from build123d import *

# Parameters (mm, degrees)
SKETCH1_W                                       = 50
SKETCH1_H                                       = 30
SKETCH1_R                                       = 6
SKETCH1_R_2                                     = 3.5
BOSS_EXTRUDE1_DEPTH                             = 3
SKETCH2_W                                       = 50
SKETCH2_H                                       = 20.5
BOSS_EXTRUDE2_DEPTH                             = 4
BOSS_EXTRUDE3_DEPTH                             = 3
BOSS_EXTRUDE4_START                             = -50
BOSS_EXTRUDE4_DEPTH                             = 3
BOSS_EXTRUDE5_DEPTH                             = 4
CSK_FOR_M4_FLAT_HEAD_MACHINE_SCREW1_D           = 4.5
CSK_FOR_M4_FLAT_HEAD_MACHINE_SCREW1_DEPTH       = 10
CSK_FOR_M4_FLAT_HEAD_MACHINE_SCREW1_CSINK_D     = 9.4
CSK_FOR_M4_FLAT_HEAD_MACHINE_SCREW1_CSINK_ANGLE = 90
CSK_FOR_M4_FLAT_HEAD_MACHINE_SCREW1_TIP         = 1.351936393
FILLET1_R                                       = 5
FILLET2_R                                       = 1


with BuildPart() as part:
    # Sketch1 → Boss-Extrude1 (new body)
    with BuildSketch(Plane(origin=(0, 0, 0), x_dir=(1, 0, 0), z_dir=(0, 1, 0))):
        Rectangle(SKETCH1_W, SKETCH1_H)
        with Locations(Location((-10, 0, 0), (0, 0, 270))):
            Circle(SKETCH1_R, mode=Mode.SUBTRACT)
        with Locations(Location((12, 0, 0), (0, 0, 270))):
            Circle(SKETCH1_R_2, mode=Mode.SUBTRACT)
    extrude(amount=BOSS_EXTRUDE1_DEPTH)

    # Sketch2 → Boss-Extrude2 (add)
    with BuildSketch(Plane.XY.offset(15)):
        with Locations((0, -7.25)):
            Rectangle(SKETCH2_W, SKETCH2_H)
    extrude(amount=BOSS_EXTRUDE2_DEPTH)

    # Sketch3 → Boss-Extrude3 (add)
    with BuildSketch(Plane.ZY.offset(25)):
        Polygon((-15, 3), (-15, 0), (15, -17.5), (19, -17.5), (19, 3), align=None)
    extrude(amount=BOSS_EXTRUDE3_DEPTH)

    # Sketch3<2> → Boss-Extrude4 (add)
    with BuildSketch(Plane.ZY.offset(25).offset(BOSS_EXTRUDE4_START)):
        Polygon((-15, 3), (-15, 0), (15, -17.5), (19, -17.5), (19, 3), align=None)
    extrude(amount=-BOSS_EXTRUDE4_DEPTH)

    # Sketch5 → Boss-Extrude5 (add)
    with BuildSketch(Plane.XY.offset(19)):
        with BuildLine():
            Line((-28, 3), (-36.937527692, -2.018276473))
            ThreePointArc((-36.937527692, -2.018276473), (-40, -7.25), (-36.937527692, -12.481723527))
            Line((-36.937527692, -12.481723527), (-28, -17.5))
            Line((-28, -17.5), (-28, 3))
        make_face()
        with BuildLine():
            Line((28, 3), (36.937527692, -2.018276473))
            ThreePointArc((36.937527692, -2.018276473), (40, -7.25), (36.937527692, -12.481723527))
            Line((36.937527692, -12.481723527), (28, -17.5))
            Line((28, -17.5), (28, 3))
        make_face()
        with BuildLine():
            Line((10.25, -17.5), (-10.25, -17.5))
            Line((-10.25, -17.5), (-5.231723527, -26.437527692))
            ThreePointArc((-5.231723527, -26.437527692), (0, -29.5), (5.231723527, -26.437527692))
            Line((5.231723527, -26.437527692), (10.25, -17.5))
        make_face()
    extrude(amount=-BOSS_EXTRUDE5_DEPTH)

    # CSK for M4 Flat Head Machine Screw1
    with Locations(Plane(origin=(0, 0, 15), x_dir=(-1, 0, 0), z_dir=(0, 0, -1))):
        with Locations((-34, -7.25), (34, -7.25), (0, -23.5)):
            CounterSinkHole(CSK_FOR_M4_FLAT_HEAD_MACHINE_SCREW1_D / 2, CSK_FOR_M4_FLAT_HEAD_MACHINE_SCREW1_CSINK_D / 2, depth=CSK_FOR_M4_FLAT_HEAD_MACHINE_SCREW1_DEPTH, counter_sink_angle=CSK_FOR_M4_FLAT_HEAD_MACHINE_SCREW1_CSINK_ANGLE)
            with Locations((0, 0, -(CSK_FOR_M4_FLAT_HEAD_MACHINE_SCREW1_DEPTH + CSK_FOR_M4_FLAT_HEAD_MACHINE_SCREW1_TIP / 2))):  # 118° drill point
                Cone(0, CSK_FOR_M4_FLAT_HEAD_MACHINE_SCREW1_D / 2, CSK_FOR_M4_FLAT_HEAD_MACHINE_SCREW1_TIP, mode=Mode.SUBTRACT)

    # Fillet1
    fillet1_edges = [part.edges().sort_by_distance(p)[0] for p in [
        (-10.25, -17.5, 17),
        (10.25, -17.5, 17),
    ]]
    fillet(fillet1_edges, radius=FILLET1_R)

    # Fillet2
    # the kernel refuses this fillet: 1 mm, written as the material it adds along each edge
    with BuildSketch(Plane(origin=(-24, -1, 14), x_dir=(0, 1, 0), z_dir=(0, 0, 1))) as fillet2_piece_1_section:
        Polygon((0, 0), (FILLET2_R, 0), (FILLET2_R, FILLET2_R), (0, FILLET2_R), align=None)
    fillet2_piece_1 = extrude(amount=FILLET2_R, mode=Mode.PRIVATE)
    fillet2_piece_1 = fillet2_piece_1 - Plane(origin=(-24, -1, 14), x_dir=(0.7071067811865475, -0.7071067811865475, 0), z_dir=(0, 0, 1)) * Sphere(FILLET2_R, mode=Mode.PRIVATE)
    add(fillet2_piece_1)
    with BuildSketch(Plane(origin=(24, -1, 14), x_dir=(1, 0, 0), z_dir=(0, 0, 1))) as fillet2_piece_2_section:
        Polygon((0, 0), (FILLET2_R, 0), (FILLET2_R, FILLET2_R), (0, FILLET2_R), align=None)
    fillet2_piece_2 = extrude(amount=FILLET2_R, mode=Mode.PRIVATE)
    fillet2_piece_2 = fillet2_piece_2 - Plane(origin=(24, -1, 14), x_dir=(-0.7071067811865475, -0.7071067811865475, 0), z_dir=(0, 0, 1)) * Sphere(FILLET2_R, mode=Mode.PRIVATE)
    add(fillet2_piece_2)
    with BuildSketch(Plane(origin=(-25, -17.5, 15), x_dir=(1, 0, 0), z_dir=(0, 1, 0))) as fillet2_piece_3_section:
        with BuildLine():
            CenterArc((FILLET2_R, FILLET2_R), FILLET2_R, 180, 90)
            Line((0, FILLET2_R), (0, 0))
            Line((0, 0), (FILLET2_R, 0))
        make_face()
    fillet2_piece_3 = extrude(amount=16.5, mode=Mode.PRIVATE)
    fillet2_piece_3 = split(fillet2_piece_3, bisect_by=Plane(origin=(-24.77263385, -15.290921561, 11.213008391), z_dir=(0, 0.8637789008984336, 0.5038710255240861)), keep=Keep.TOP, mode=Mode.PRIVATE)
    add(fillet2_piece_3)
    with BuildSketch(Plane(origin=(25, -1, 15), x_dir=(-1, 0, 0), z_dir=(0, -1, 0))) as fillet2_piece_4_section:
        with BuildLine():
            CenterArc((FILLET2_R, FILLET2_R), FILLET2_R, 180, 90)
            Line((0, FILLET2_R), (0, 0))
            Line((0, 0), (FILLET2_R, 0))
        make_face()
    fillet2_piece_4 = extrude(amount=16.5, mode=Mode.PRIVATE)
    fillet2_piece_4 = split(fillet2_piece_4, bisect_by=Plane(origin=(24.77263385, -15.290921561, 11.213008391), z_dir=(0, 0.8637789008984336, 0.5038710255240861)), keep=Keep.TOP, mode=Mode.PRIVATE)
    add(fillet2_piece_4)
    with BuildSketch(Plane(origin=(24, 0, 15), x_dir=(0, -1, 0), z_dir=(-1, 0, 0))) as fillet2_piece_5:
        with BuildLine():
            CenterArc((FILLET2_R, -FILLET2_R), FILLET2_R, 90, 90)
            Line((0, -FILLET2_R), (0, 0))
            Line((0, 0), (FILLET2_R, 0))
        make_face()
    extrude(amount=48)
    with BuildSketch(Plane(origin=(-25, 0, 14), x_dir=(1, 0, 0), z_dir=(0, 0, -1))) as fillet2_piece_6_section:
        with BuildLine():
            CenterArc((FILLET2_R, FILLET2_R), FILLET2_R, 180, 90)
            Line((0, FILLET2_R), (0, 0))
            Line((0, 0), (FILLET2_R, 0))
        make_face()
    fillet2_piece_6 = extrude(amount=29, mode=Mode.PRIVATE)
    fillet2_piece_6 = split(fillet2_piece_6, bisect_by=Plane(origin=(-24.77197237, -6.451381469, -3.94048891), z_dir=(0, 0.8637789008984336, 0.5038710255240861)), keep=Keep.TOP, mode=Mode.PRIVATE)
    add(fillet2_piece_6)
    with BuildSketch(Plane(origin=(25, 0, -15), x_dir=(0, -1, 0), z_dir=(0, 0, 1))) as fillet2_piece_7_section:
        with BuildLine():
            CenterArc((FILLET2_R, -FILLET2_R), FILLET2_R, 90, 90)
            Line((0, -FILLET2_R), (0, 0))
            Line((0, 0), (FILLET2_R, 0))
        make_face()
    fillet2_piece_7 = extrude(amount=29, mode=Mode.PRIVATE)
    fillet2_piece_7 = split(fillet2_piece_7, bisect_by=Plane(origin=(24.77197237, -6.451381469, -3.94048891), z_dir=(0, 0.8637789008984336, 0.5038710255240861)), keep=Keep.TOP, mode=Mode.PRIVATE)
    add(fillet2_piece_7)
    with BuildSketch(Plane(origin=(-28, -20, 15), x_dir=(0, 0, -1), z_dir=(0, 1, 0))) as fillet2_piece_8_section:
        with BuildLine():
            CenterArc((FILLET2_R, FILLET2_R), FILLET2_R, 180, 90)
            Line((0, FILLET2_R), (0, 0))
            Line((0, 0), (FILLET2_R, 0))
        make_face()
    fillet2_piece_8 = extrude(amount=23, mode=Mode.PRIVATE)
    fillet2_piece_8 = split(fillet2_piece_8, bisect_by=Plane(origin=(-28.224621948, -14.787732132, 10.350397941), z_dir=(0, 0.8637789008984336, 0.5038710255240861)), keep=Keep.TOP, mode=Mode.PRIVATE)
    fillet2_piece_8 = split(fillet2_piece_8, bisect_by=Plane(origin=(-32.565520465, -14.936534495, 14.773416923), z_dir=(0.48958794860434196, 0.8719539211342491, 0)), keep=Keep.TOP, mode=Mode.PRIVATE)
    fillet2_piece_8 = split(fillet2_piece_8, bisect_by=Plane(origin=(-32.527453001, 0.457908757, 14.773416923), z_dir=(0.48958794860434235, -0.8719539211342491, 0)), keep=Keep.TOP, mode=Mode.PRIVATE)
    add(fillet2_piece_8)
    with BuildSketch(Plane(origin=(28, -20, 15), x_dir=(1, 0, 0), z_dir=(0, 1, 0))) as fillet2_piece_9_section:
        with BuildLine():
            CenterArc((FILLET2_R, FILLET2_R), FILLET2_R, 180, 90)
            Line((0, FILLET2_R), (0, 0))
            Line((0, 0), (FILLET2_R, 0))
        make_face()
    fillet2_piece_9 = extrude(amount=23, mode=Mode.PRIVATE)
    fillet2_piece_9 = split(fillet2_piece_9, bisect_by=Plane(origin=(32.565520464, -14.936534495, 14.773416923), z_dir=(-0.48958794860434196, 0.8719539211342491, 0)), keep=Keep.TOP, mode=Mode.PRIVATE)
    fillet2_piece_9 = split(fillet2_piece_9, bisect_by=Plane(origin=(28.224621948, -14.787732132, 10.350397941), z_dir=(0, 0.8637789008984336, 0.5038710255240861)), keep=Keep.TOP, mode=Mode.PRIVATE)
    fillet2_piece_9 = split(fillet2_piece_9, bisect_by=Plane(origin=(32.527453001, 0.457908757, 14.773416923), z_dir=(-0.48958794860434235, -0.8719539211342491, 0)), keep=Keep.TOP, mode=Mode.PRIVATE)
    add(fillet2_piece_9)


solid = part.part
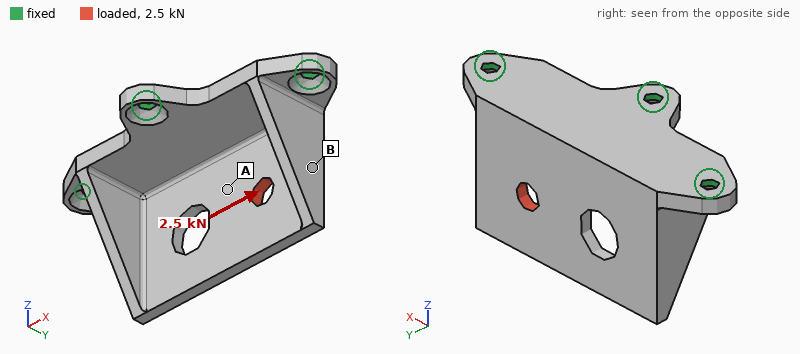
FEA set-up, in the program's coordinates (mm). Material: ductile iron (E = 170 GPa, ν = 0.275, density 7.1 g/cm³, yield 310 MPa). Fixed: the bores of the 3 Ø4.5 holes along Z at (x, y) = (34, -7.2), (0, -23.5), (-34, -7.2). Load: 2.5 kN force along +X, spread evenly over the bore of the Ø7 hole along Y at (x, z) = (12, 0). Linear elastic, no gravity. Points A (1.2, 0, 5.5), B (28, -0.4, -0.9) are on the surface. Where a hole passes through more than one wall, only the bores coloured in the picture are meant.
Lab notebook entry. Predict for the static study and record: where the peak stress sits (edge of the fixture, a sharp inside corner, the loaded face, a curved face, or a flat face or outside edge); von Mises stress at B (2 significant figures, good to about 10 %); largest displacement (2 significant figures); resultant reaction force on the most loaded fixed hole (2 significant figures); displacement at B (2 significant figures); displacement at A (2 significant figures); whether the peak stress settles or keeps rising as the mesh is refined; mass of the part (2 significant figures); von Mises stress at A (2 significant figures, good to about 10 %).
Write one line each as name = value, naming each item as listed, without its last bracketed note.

where the peak stress sits = edge of the fixture
von Mises stress at B = 23 MPa
largest displacement = 51 µm
resultant reaction force on the most loaded fixed hole = 1.4 kN
displacement at B = 28 µm
displacement at A = 11 µm
whether the peak stress settles or keeps rising as the mesh is refined = keeps rising
mass of the part = 88 g
von Mises stress at A = 56 MPa
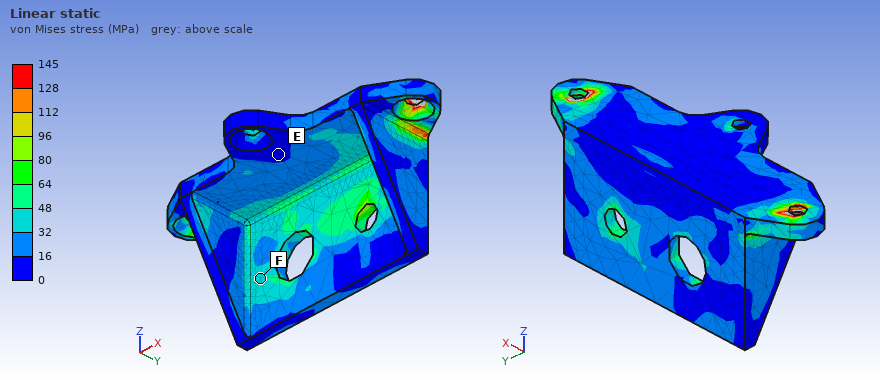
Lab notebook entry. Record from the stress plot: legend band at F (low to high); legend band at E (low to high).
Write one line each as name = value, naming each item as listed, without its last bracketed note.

legend band at F = 32 to 48 MPa
legend band at E = 0 to 16 MPa
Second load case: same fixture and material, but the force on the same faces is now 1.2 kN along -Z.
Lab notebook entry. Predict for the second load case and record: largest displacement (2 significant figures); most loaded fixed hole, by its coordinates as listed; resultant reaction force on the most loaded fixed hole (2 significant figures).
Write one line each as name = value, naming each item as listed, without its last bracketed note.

largest displacement = 85 µm
most loaded fixed hole, by its coordinates as listed = (34, -7.2)
resultant reaction force on the most loaded fixed hole = 1.1 kN
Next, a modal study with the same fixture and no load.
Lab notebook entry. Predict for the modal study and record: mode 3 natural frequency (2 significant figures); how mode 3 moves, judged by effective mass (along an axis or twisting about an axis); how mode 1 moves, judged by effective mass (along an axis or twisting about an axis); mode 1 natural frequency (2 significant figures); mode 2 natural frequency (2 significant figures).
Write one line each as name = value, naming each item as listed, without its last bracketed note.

mode 3 natural frequency = 6800 Hz
how mode 3 moves, judged by effective mass = along Z
how mode 1 moves, judged by effective mass = along Y
mode 1 natural frequency = 2600 Hz
mode 2 natural frequency = 4500 Hz
